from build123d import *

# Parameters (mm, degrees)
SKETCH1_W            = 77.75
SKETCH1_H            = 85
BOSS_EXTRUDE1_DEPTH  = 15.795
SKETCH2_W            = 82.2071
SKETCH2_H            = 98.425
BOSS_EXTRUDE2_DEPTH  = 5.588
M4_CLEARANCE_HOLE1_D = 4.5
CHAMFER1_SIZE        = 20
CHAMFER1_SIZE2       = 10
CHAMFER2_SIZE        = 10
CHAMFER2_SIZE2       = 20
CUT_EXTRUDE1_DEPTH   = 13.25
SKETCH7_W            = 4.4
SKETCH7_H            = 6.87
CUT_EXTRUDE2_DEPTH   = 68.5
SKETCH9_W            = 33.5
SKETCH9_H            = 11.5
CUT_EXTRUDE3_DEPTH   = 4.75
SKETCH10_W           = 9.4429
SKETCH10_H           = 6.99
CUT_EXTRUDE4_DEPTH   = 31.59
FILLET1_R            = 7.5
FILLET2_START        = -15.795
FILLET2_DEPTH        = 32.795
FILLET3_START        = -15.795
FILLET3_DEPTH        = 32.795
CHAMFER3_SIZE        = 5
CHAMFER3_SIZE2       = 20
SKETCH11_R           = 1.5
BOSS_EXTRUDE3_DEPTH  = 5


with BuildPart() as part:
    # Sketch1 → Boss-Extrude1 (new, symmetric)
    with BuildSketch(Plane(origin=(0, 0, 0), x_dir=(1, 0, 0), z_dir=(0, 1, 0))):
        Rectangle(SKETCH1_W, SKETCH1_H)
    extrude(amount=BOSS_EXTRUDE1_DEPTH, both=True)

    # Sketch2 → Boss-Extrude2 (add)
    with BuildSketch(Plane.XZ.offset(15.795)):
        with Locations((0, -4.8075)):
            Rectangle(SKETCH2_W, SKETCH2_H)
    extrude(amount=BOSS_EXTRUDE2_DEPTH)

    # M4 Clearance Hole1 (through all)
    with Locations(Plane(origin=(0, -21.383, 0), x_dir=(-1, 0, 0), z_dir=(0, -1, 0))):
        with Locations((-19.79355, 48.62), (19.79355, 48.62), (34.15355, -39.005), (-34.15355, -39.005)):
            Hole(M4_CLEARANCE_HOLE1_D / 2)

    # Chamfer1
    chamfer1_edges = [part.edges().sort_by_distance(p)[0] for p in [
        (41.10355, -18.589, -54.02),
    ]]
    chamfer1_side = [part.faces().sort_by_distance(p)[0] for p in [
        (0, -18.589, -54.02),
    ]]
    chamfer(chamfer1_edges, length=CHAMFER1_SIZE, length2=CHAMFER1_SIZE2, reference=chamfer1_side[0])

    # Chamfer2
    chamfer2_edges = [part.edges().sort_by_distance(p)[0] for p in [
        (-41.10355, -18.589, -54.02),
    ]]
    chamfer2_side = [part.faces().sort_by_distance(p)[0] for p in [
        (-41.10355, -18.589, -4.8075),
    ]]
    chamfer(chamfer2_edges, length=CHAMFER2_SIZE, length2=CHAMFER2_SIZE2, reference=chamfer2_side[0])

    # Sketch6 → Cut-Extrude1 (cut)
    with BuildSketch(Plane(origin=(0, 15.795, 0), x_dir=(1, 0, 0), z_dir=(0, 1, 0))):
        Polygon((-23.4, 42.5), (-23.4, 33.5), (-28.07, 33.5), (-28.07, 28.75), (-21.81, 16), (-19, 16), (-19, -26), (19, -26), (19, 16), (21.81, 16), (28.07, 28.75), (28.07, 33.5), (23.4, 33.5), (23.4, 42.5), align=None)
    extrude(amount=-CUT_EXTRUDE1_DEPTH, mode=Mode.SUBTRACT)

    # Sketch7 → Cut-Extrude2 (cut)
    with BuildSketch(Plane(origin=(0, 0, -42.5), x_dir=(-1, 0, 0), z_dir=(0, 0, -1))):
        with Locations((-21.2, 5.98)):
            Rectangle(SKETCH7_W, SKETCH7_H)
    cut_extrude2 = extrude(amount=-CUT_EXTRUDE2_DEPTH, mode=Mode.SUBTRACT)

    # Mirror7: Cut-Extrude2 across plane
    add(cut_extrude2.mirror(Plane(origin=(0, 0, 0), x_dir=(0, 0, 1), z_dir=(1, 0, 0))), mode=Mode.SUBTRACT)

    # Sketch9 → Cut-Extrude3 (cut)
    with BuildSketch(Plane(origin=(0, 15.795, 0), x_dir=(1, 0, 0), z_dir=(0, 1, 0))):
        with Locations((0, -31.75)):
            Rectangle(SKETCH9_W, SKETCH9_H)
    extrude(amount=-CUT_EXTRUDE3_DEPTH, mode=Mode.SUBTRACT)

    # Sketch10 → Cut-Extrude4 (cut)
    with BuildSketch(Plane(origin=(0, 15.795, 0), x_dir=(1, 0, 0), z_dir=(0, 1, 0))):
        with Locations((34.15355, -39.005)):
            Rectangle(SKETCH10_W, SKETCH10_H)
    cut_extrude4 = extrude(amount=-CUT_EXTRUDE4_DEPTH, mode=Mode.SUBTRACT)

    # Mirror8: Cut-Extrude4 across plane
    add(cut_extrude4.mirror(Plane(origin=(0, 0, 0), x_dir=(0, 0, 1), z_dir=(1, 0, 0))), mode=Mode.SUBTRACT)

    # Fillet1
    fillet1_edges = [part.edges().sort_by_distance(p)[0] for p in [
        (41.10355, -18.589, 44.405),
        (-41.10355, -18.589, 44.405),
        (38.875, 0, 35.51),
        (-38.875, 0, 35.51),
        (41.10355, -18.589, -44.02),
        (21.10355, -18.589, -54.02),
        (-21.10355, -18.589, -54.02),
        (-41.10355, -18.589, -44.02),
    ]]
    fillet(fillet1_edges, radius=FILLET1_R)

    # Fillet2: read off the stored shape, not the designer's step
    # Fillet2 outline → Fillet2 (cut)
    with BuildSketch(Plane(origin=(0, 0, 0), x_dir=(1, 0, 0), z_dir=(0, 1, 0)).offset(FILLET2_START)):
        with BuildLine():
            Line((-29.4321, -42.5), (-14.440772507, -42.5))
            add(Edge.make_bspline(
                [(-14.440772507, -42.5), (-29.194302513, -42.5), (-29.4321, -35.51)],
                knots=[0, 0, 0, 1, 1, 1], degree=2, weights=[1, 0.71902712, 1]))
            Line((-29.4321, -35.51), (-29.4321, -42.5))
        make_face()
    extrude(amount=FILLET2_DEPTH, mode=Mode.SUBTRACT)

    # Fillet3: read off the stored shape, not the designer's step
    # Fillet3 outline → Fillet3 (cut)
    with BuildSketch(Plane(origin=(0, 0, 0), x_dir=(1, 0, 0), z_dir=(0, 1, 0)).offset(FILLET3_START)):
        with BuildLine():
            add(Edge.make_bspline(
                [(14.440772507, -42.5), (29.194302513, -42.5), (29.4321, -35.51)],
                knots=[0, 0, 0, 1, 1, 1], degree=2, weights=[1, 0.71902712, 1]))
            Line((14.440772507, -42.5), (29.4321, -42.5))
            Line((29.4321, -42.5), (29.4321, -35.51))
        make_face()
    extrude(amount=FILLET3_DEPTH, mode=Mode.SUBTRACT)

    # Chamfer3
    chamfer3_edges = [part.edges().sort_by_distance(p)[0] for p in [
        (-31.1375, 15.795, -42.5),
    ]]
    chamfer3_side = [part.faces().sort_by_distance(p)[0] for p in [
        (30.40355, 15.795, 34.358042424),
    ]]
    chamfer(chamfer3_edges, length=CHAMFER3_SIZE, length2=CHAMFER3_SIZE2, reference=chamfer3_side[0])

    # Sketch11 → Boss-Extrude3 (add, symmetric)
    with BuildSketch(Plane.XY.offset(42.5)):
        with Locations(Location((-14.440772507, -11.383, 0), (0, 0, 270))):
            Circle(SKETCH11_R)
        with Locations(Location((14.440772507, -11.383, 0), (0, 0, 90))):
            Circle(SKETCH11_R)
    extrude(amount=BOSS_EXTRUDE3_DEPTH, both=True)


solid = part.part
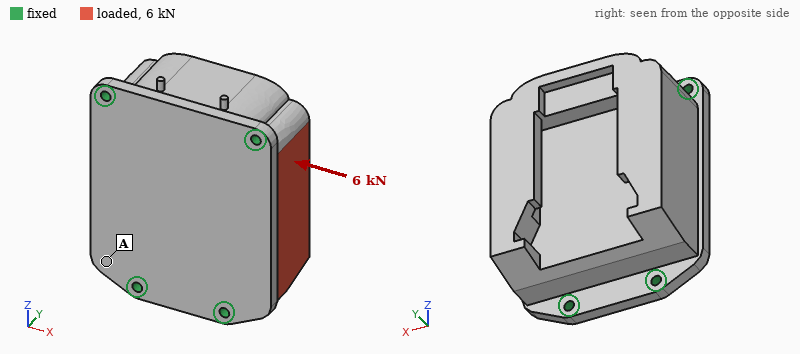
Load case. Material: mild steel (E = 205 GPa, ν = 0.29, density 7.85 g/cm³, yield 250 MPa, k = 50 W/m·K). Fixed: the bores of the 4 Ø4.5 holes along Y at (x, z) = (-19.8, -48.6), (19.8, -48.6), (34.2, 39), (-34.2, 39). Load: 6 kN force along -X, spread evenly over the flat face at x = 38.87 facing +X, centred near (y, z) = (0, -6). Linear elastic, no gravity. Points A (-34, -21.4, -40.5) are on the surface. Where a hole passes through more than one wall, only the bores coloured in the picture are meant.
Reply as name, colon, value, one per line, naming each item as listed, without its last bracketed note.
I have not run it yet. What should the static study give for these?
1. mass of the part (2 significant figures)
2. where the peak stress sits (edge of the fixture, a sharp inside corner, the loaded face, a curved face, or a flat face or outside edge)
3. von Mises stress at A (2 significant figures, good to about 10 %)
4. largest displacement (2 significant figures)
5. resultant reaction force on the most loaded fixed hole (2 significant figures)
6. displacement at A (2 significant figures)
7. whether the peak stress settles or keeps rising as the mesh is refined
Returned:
mass of the part: 1.6 kg
where the peak stress sits: edge of the fixture
von Mises stress at A: 10 MPa
largest displacement: 8.8 µm
resultant reaction force on the most loaded fixed hole: 2.4 kN
displacement at A: 2.5 µm
whether the peak stress settles or keeps rising as the mesh is refined: keeps rising
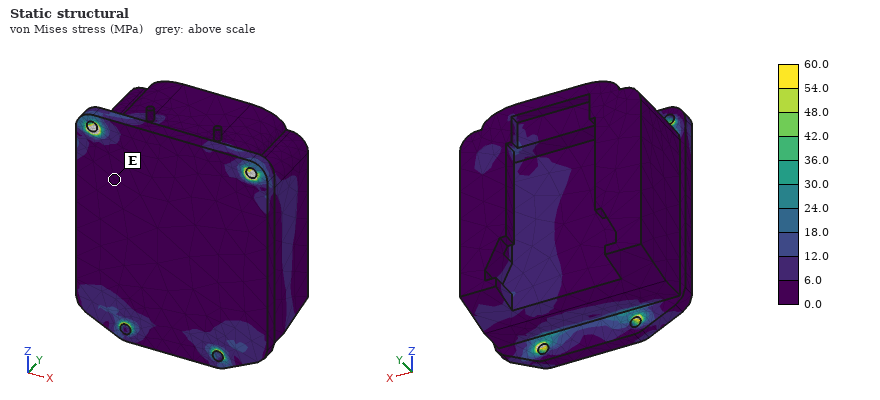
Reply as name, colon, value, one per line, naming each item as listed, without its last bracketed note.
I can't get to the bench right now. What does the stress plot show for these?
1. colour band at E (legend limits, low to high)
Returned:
colour band at E: 0.0 to 6.0 MPa
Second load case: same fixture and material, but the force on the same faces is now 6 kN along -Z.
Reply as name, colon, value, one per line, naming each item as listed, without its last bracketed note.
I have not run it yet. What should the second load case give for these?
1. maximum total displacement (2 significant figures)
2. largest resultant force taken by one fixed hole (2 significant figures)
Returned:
maximum total displacement: 4.7 µm
largest resultant force taken by one fixed hole: 2.5 kN
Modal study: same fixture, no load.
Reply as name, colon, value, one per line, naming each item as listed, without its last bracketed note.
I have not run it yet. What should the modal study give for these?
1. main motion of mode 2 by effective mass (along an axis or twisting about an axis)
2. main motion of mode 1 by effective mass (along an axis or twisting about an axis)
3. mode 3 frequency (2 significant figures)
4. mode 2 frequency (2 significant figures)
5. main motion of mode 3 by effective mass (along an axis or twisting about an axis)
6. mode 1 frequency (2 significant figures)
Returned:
main motion of mode 2 by effective mass: along Y
main motion of mode 1 by effective mass: along X
mode 3 frequency: 7400 Hz
mode 2 frequency: 5300 Hz
main motion of mode 3 by effective mass: along Z
mode 1 frequency: 5000 Hz
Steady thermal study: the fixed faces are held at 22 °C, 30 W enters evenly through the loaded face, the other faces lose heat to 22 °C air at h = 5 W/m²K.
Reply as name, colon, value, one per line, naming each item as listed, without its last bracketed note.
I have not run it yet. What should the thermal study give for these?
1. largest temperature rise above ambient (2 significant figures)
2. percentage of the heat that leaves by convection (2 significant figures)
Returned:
largest temperature rise above ambient: 24 K
percentage of the heat that leaves by convection: 5.8 %
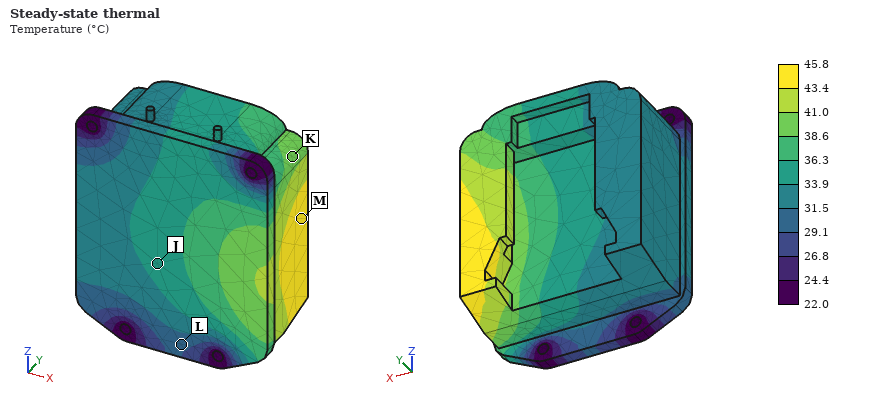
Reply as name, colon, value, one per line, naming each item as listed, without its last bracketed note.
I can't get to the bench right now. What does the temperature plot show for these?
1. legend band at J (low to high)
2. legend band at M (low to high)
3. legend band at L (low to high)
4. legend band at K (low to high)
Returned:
legend band at J: 33.9 to 36.3 °C
legend band at M: 43.4 to 45.8 °C
legend band at L: 29.1 to 31.5 °C
legend band at K: 38.6 to 41.0 °C
